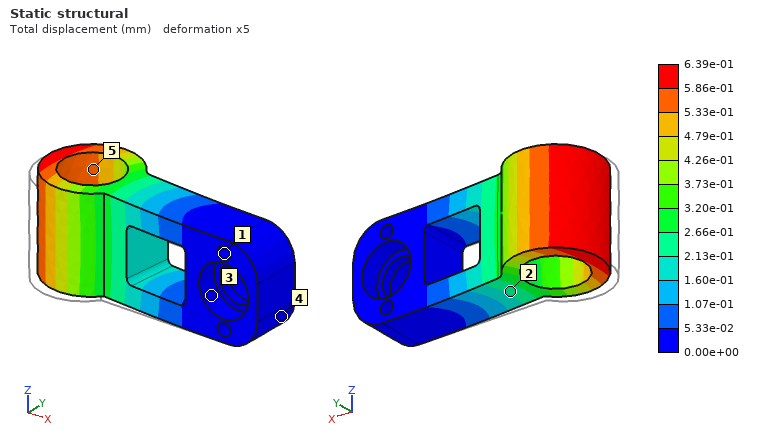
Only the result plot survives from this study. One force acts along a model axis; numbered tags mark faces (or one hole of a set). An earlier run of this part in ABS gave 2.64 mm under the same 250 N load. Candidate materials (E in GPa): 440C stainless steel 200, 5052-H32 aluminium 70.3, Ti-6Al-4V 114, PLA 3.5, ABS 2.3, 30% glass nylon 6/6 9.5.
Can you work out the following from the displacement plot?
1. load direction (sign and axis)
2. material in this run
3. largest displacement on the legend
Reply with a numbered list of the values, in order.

1. +Y
2. 30% glass nylon 6/6
3. 6.39e-01 mm
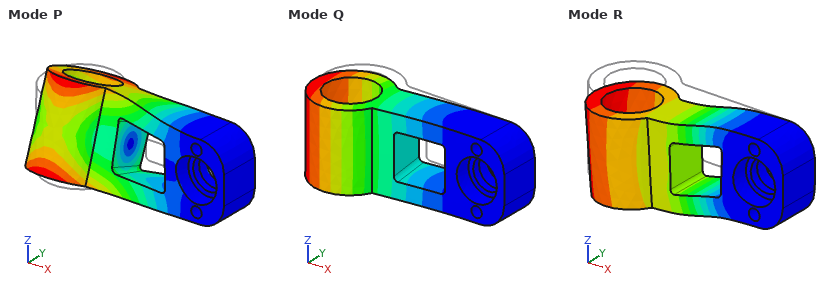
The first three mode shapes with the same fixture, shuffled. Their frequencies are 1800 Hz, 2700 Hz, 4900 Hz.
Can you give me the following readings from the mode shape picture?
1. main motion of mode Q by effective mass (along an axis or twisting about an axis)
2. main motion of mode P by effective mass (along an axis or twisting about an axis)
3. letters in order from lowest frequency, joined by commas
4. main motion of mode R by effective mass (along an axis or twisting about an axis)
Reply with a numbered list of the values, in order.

1. along Y
2. twisting about X
3. Q, R, P
4. along Z
